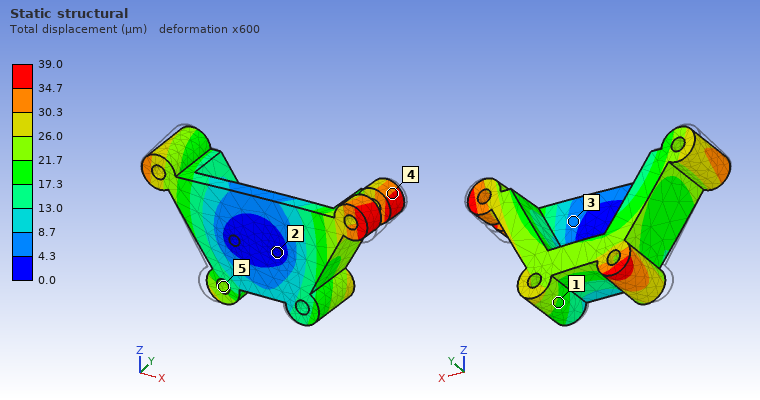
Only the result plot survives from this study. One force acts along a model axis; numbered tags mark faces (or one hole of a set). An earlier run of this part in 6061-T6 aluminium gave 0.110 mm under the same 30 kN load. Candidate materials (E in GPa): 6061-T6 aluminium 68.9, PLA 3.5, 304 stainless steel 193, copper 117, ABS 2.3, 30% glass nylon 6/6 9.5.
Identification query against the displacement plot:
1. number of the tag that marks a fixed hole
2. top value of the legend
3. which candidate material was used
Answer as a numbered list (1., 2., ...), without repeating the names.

1. 2
2. 39.0 µm
3. 304 stainless steel
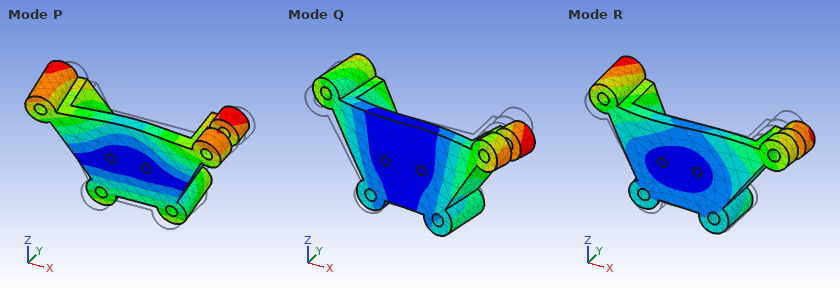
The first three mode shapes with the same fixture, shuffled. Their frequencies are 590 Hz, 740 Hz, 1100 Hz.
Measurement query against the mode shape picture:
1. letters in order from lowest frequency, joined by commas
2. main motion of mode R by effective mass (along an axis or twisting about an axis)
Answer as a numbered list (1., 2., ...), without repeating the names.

1. P, Q, R
2. twisting about Y
